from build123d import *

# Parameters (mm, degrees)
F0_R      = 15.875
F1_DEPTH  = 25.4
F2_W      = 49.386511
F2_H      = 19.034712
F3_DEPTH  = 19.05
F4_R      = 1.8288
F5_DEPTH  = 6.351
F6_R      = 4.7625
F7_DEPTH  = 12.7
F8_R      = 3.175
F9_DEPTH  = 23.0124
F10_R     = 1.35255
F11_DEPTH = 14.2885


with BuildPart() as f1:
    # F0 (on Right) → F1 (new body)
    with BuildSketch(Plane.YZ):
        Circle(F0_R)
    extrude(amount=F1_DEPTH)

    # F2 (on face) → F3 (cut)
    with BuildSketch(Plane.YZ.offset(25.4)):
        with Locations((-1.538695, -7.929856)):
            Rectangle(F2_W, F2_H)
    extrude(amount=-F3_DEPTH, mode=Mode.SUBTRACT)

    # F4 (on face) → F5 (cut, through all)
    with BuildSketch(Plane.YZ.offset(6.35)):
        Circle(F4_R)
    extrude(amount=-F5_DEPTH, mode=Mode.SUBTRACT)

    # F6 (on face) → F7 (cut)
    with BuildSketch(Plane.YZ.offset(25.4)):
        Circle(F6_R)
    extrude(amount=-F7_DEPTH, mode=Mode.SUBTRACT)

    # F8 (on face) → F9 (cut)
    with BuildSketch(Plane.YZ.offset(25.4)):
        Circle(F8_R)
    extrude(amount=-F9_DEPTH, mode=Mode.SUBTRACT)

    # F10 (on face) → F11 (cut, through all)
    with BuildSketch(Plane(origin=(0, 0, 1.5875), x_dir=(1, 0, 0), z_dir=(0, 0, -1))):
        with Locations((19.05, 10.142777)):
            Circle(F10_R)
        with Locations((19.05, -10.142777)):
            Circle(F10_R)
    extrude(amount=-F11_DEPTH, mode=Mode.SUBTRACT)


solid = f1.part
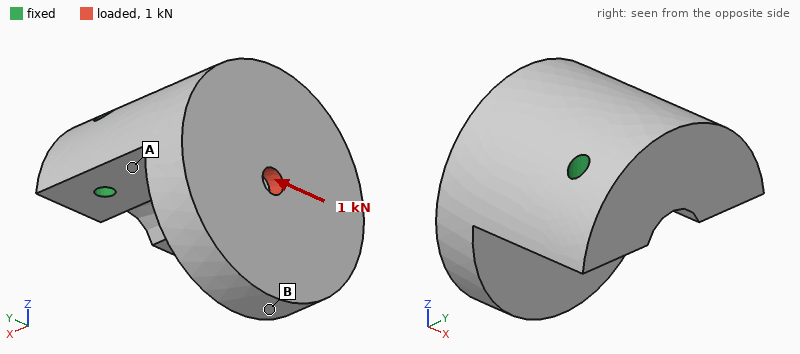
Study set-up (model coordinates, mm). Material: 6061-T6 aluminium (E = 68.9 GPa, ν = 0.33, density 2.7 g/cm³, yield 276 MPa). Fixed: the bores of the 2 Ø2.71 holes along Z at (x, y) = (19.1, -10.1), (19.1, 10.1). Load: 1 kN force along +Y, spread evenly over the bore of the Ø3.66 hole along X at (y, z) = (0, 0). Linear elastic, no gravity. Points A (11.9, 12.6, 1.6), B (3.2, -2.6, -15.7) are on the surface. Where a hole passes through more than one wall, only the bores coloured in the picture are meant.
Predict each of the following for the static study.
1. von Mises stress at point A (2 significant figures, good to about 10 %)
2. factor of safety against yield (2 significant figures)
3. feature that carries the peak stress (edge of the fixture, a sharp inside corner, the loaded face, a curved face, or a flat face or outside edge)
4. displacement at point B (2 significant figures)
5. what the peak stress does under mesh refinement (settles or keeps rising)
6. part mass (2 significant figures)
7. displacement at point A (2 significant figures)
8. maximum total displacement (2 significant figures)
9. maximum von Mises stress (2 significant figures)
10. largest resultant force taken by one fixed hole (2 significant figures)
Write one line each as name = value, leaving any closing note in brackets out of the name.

von Mises stress at point A = 12 MPa
factor of safety against yield = 4.1
feature that carries the peak stress = the loaded face
displacement at point B = 13 µm
what the peak stress does under mesh refinement = settles
part mass = 30 g
displacement at point A = 3.3 µm
maximum total displacement = 13 µm
maximum von Mises stress = 67 MPa
largest resultant force taken by one fixed hole = 1.0 kN
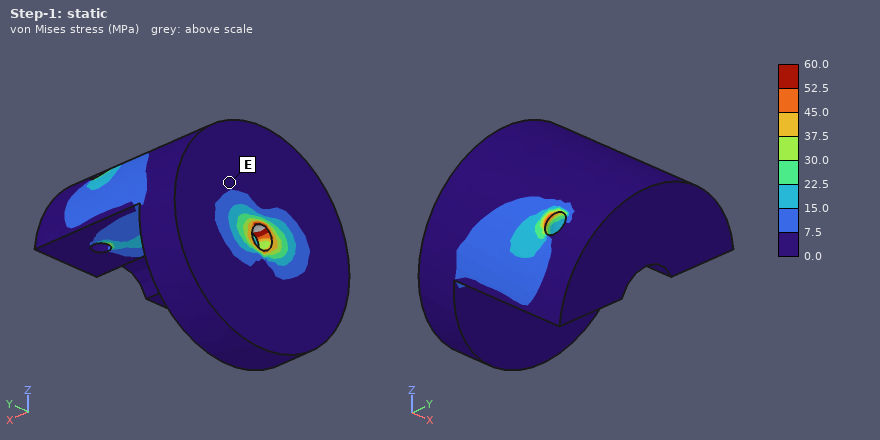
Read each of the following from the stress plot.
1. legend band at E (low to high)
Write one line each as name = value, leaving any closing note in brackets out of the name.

legend band at E = 0.0 to 7.5 MPa
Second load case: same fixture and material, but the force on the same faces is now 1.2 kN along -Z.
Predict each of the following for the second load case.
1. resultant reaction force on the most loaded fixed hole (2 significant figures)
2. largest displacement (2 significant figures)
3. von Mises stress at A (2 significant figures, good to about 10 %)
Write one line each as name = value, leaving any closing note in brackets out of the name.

resultant reaction force on the most loaded fixed hole = 620 N
largest displacement = 38 µm
von Mises stress at A = 22 MPa
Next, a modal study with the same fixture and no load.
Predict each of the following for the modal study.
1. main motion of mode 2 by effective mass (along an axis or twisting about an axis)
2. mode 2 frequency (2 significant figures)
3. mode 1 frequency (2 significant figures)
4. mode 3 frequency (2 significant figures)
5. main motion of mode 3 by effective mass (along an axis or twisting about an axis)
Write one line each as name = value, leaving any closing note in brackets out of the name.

main motion of mode 2 by effective mass = along Y
mode 2 frequency = 13 kHz
mode 1 frequency = 8800 Hz
mode 3 frequency = 17 kHz
main motion of mode 3 by effective mass = along Z
